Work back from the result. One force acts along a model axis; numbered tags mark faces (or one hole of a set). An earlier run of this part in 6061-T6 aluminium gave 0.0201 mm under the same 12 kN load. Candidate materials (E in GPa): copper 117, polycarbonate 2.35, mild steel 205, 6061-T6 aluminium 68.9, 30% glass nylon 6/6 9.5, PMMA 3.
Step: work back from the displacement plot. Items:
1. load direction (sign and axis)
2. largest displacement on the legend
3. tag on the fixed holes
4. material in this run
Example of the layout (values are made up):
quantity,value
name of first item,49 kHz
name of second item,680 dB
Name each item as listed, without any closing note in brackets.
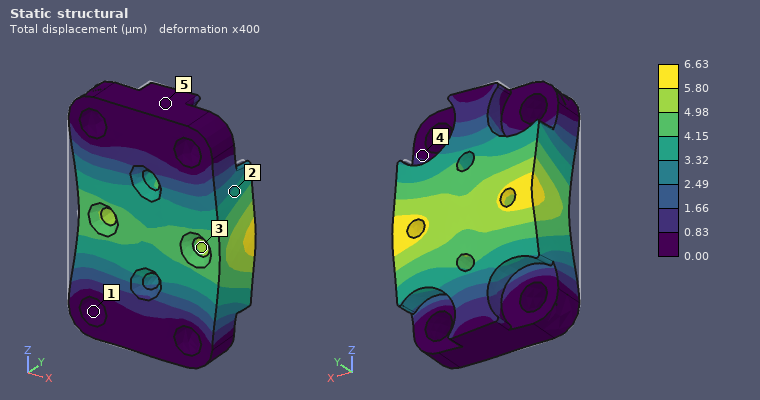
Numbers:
quantity,value
load direction,+X
largest displacement on the legend,6.63 µm
tag on the fixed holes,1
material in this run,mild steel
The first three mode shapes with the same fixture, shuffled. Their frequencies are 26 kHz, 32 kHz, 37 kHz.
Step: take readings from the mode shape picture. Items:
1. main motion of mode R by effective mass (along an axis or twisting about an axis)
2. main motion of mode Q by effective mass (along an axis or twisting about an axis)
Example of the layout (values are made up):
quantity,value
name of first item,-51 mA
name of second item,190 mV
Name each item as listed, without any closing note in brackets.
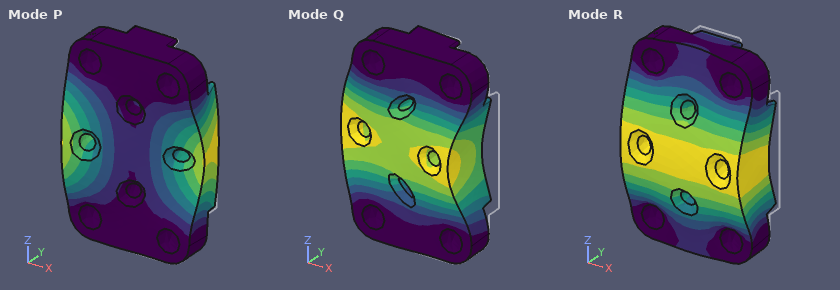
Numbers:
quantity,value
main motion of mode R by effective mass,along Y
main motion of mode Q by effective mass,along X
